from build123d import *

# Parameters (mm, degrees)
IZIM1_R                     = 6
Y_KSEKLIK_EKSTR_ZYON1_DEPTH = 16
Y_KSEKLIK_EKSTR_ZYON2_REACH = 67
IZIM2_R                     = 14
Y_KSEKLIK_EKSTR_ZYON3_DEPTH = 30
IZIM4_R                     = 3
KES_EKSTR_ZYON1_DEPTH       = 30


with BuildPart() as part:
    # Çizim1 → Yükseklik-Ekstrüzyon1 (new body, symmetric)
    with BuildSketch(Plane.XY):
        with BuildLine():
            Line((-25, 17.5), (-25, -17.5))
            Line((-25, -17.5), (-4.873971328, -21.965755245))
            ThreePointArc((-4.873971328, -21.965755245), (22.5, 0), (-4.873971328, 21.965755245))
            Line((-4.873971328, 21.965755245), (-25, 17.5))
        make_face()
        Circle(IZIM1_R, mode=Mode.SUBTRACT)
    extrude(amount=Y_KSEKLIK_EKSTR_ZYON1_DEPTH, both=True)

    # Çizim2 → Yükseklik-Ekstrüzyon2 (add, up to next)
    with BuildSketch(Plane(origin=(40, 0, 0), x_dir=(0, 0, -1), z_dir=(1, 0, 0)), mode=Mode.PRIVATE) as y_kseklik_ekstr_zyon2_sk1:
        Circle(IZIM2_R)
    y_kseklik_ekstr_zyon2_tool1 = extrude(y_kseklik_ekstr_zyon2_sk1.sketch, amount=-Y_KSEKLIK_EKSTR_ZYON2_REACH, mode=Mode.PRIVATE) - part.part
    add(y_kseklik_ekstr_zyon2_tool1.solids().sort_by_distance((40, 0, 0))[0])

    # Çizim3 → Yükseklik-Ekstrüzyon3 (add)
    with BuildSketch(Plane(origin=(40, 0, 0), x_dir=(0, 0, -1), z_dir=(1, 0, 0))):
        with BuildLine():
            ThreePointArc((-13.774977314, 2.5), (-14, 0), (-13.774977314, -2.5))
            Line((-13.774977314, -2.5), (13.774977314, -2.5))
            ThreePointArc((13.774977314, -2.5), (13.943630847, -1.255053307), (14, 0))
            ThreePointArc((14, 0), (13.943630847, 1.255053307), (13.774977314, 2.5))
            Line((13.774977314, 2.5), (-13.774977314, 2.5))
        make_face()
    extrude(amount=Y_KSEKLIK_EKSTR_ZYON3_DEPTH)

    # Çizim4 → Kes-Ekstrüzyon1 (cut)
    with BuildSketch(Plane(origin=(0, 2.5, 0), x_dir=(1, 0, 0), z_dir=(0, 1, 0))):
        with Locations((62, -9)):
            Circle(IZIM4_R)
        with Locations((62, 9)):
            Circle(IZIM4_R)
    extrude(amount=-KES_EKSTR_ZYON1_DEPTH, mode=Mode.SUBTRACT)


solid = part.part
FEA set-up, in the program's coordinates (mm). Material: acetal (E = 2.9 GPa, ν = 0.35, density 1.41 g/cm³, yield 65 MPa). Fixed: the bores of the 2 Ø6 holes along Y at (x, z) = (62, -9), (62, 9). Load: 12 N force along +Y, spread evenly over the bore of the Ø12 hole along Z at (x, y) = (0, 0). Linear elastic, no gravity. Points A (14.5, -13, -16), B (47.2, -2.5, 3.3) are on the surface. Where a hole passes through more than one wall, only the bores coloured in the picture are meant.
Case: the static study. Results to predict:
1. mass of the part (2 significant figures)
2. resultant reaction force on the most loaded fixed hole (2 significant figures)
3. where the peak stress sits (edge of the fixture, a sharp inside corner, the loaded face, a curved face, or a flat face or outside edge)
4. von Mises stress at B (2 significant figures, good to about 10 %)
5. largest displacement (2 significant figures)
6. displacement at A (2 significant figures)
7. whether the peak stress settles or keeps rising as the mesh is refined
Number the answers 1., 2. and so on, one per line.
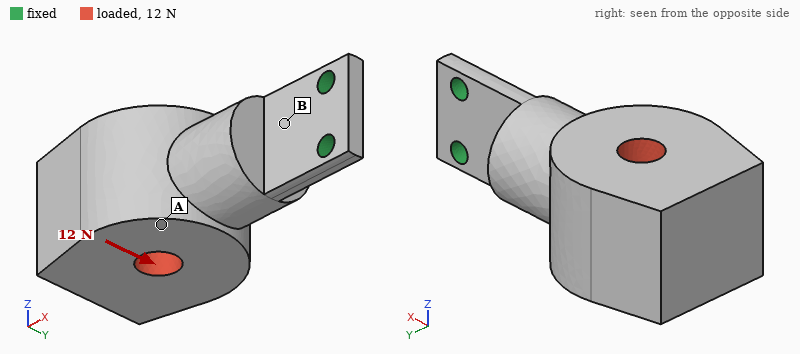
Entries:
1. 98 g
2. 6.0 N
3. edge of the fixture
4. 4.4 MPa
5. 1.1 mm
6. 0.56 mm
7. keeps rising
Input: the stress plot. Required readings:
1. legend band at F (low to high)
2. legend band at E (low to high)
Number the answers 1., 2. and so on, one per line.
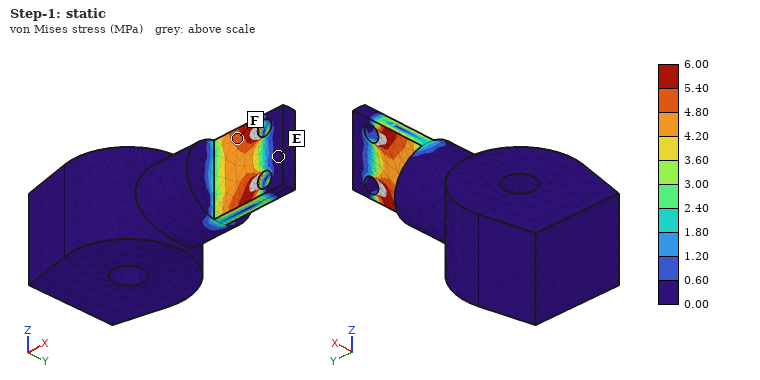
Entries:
1. 4.80 to 5.40 MPa
2. 0.00 to 0.60 MPa
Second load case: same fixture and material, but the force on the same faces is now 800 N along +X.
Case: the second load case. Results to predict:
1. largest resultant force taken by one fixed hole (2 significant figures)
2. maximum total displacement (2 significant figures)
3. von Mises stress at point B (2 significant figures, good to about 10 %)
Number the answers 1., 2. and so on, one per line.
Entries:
1. 410 N
2. 68 µm
3. 5.7 MPa
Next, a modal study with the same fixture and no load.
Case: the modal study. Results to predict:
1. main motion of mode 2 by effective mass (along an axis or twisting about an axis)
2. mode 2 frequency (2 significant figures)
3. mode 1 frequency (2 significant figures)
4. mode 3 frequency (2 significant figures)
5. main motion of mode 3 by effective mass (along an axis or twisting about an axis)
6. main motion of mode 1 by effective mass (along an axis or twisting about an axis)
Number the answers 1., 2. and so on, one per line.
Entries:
1. along Z
2. 320 Hz
3. 65 Hz
4. 370 Hz
5. twisting about X
6. along Y
